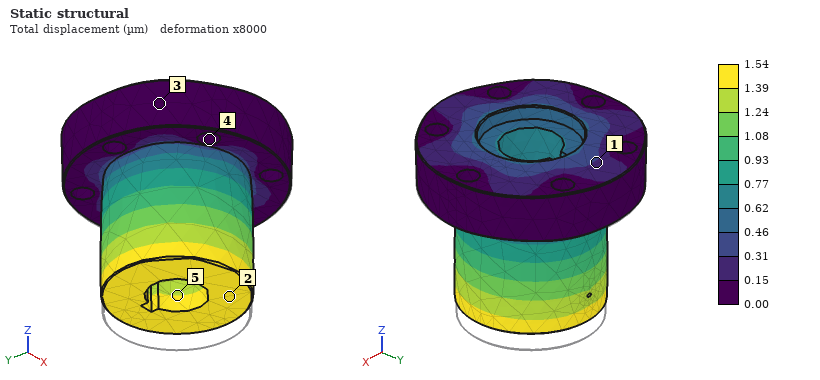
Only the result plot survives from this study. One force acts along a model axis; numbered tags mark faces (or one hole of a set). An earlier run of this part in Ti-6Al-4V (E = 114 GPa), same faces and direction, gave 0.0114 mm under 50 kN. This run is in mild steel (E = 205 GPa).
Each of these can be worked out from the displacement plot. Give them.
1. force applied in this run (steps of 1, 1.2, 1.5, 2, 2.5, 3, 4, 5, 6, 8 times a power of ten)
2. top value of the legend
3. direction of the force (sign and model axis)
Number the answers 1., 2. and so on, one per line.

1. 12 kN
2. 1.54 µm
3. +Z
